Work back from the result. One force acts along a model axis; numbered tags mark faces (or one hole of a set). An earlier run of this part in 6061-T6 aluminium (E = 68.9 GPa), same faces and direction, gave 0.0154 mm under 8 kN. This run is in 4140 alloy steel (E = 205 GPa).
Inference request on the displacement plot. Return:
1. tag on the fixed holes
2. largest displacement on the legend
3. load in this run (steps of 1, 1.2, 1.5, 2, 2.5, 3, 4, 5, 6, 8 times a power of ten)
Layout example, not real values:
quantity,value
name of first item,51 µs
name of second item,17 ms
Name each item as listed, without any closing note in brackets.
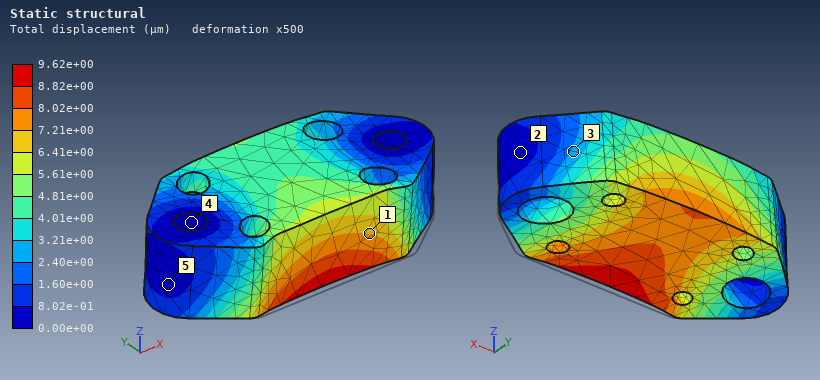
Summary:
quantity,value
tag on the fixed holes,4
largest displacement on the legend,9.62e+00 µm
load in this run,15 kN
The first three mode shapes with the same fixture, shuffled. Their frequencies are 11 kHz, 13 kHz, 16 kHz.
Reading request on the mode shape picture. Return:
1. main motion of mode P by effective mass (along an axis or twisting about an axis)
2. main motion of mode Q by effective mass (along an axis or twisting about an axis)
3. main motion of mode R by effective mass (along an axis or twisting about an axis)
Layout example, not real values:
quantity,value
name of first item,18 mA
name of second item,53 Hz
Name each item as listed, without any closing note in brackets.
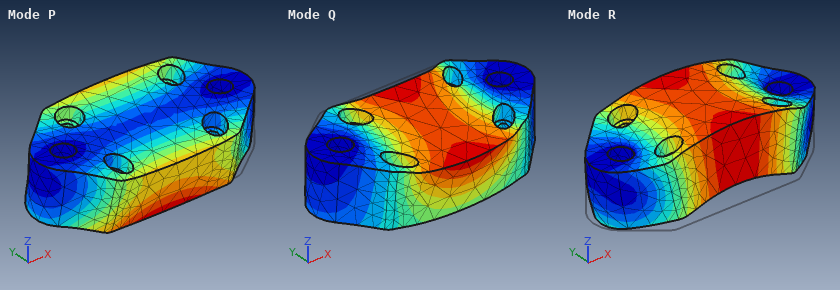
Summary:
quantity,value
main motion of mode P by effective mass,along Y
main motion of mode Q by effective mass,along Y
main motion of mode R by effective mass,along Z
